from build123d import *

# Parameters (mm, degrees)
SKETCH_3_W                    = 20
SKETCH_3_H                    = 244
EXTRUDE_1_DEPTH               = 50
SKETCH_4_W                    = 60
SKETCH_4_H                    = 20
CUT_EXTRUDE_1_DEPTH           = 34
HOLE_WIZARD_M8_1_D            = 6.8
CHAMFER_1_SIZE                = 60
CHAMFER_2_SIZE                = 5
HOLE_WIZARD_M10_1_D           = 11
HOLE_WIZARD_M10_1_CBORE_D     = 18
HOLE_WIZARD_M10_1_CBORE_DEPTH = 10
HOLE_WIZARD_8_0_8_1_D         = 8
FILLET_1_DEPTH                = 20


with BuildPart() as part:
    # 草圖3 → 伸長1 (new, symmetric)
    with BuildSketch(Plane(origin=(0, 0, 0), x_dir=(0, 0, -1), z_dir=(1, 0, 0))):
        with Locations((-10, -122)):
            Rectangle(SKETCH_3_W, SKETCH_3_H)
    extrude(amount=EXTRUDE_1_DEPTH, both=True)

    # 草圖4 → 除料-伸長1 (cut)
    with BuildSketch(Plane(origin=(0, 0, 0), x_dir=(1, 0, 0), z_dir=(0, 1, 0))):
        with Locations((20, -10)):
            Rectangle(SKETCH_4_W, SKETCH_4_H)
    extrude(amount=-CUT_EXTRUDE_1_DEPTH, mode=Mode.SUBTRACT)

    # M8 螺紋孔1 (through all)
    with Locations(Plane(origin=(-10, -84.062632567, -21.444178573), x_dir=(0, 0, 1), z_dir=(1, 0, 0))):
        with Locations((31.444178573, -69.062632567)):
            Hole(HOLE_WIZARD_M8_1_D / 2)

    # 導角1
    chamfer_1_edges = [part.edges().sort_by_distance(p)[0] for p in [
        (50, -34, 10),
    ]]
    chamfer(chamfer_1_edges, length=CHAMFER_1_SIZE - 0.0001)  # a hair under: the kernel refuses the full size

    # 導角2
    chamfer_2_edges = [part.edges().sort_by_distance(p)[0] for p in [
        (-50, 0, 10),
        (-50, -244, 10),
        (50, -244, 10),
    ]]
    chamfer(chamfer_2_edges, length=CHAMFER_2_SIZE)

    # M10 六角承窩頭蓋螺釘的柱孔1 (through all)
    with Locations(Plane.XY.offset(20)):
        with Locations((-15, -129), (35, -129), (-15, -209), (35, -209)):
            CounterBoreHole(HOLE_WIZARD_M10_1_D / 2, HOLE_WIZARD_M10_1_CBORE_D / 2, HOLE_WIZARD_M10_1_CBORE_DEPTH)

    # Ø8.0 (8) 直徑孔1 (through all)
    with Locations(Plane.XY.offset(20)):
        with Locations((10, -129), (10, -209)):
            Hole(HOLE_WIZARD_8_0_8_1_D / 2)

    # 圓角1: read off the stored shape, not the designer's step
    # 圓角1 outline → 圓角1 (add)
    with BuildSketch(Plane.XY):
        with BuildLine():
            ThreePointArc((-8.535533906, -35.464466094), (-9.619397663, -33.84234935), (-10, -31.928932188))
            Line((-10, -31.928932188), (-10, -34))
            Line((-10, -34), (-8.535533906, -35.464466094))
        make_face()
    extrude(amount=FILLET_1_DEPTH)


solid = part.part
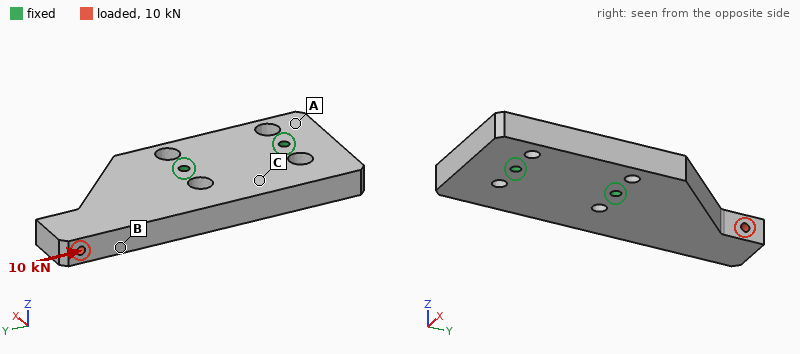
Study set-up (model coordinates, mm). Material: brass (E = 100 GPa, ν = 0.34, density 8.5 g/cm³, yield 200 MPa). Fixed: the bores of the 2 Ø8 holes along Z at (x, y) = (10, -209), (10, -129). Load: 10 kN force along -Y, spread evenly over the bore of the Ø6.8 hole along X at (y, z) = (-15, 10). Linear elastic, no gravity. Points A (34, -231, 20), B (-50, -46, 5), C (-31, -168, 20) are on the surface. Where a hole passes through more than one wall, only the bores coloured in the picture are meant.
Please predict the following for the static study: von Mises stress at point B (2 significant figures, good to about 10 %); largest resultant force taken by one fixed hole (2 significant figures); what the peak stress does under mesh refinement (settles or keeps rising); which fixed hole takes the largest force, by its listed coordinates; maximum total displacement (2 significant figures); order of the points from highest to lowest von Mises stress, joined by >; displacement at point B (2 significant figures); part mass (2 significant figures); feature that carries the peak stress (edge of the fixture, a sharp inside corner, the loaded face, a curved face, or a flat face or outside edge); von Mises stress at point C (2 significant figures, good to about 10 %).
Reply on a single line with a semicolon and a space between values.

14 MPa; 8.0 kN; keeps rising; (10, -129); 49 µm; B > C > A; 34 µm; 3.3 kg; edge of the fixture; 7.4 MPa
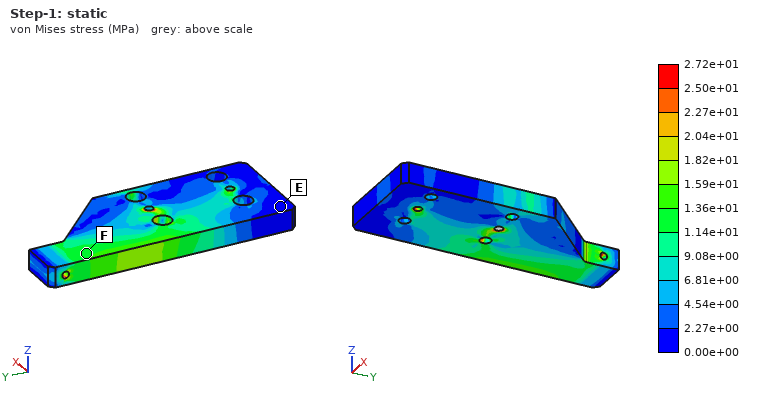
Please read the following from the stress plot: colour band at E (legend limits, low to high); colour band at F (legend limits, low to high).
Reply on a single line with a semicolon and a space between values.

0.00e+00 to 2.27e+00 MPa; 1.14e+01 to 1.36e+01 MPa
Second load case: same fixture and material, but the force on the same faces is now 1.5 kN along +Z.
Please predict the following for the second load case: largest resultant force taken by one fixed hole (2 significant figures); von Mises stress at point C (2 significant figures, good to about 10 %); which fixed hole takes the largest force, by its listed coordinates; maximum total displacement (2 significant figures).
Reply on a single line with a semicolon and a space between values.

2.5 kN; 7.5 MPa; (10, -129); 0.26 mm
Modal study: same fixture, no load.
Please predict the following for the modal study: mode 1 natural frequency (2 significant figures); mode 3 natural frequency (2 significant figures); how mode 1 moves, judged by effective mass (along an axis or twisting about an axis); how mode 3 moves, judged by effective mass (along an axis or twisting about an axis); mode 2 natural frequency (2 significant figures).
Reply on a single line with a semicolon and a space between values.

720 Hz; 2000 Hz; along Z; along X; 1900 Hz
